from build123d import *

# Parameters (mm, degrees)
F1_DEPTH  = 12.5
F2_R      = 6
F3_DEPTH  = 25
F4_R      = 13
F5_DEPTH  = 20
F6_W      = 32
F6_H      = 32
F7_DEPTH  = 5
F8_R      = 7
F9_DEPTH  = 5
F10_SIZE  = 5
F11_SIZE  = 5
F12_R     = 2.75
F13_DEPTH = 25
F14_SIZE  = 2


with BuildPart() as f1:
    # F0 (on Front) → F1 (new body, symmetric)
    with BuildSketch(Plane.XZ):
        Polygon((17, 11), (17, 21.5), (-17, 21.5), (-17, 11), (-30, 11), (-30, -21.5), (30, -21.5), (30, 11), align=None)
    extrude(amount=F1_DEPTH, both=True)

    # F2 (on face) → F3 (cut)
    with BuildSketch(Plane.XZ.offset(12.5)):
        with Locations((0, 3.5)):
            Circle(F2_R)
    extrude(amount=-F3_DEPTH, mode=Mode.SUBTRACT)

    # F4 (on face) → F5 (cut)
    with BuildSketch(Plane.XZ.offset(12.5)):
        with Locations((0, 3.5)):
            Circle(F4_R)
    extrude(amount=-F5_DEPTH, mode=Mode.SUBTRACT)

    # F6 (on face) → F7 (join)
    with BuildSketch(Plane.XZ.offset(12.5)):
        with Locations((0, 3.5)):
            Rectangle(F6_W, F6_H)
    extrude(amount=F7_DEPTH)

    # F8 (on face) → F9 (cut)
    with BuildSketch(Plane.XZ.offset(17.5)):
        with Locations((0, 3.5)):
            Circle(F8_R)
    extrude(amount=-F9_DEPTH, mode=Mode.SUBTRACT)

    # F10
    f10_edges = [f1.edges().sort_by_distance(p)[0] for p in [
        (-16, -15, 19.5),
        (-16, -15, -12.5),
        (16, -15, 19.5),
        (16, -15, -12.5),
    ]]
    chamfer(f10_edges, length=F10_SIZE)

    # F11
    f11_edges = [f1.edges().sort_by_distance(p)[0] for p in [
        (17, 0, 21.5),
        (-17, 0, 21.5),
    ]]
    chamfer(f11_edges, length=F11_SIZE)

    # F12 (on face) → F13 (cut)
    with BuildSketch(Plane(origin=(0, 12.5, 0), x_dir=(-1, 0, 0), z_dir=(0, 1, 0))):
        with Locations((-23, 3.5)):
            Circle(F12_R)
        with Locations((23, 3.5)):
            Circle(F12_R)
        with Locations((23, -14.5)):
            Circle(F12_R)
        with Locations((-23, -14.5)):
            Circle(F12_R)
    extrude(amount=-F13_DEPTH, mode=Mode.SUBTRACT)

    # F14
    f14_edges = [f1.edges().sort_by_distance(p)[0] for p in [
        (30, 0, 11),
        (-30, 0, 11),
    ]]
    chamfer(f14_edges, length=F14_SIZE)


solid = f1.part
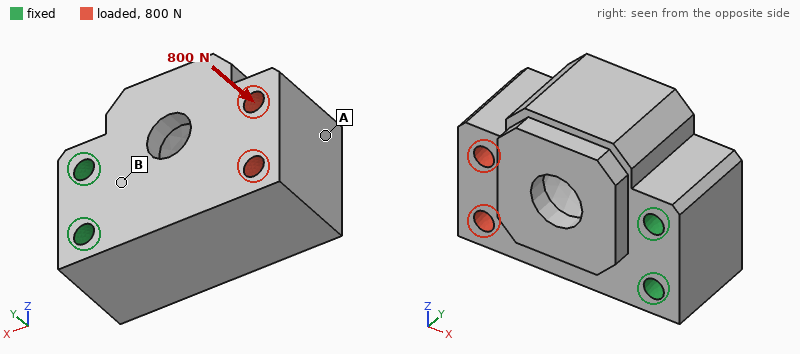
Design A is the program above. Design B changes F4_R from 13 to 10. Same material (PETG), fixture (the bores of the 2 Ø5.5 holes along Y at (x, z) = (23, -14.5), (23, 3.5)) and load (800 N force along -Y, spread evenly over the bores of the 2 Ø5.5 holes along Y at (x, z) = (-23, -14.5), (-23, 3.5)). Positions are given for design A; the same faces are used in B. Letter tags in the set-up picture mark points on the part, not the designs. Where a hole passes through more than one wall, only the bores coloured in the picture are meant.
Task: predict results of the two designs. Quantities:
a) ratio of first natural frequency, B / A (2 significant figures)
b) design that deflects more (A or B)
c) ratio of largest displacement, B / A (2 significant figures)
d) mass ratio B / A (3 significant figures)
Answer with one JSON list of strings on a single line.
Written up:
["1.1", "A", "0.87", "1.09"]
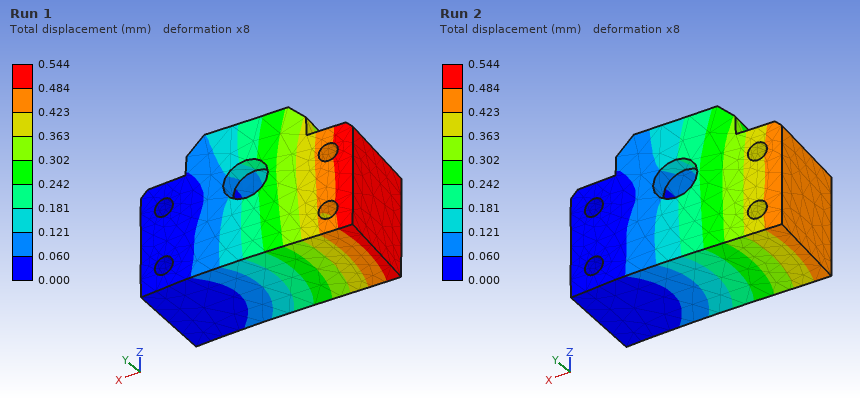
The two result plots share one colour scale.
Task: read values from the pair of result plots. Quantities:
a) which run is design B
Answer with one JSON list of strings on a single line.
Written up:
["Run 2"]
